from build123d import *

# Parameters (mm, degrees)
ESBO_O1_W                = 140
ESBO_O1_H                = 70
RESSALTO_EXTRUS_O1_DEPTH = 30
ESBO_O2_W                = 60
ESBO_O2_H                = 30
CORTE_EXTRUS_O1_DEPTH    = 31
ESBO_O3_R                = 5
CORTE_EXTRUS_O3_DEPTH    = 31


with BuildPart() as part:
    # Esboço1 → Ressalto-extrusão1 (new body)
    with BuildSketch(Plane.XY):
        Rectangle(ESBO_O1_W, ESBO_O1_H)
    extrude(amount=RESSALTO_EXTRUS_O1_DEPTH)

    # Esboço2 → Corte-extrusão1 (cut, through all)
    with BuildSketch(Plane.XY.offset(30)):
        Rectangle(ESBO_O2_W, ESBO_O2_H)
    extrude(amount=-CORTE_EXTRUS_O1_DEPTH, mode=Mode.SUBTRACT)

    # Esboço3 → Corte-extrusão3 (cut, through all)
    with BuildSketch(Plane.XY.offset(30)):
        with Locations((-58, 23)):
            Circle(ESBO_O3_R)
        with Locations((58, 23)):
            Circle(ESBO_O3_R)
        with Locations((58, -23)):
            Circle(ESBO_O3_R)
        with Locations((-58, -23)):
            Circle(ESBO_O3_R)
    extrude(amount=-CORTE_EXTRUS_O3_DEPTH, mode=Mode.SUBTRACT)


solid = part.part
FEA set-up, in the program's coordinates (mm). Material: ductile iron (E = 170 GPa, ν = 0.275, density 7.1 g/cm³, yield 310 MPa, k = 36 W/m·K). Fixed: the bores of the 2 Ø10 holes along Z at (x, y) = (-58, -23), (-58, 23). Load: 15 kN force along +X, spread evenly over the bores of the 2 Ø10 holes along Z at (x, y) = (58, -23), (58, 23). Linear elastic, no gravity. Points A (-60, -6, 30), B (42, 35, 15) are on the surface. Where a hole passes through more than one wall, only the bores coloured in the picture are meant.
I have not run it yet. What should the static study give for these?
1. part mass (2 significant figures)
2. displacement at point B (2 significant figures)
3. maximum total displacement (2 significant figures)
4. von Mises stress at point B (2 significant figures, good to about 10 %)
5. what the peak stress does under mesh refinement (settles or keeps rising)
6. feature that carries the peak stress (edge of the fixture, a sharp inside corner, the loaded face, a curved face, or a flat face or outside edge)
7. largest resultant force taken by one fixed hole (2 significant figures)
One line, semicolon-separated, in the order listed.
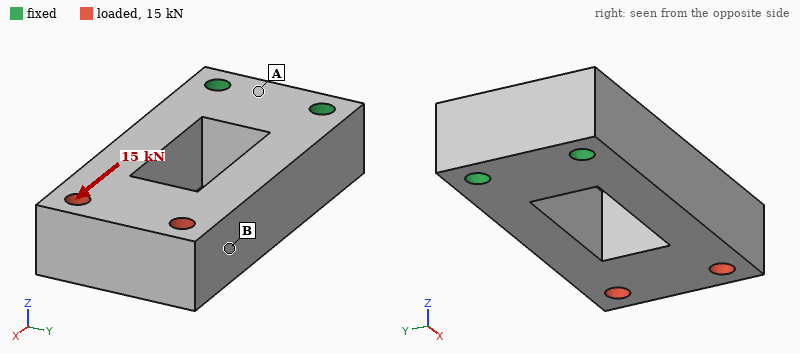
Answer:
1.6 kg; 6.7 µm; 8.8 µm; 13 MPa; keeps rising; edge of the fixture; 7.5 kN
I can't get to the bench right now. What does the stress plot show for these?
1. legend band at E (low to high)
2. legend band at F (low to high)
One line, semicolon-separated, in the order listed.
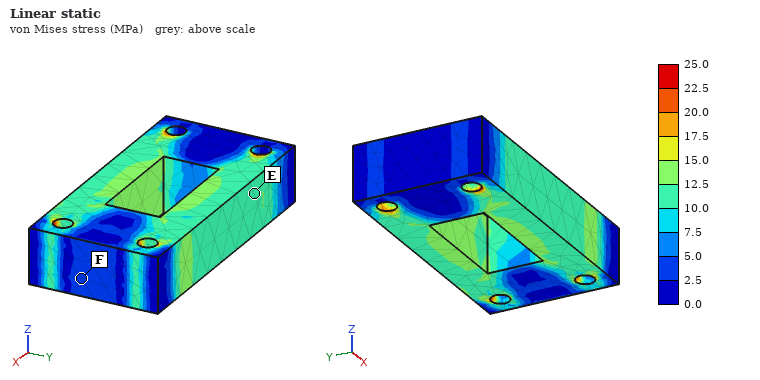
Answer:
10.0 to 12.5 MPa; 2.5 to 5.0 MPa
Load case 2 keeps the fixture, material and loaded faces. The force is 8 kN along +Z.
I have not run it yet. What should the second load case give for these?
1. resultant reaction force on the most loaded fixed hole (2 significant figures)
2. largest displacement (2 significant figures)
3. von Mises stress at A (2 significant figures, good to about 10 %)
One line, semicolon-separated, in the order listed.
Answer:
4.0 kN; 0.28 mm; 20 MPa
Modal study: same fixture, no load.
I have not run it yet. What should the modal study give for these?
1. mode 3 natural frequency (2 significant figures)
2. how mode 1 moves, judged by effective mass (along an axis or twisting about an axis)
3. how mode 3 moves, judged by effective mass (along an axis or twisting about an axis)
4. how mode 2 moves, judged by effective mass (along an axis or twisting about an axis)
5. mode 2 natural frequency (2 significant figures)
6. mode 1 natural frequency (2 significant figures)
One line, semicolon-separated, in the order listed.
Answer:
3300 Hz; along Z; twisting about X; along Y; 1900 Hz; 1200 Hz
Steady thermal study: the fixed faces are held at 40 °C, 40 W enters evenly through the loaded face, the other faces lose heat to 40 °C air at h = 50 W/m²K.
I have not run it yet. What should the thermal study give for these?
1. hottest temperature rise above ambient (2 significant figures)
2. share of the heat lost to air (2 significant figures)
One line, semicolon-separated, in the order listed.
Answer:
42 K; 71 %
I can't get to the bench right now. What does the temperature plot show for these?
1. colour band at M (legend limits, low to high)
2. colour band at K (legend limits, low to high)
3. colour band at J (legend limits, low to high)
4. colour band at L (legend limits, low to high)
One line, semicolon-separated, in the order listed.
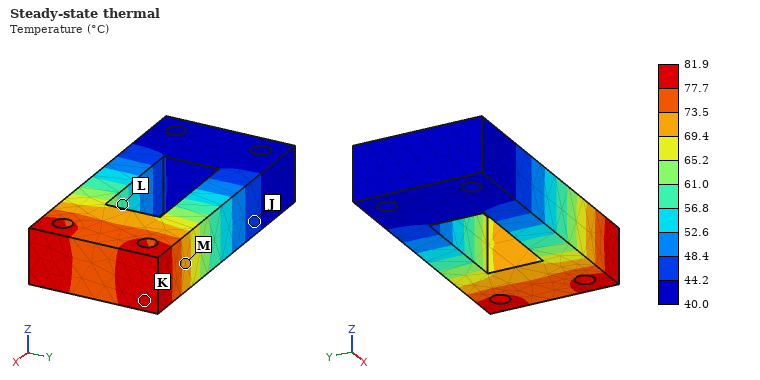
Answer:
69.4 to 73.5 °C; 77.7 to 81.9 °C; 44.2 to 48.4 °C; 56.8 to 61.0 °C
